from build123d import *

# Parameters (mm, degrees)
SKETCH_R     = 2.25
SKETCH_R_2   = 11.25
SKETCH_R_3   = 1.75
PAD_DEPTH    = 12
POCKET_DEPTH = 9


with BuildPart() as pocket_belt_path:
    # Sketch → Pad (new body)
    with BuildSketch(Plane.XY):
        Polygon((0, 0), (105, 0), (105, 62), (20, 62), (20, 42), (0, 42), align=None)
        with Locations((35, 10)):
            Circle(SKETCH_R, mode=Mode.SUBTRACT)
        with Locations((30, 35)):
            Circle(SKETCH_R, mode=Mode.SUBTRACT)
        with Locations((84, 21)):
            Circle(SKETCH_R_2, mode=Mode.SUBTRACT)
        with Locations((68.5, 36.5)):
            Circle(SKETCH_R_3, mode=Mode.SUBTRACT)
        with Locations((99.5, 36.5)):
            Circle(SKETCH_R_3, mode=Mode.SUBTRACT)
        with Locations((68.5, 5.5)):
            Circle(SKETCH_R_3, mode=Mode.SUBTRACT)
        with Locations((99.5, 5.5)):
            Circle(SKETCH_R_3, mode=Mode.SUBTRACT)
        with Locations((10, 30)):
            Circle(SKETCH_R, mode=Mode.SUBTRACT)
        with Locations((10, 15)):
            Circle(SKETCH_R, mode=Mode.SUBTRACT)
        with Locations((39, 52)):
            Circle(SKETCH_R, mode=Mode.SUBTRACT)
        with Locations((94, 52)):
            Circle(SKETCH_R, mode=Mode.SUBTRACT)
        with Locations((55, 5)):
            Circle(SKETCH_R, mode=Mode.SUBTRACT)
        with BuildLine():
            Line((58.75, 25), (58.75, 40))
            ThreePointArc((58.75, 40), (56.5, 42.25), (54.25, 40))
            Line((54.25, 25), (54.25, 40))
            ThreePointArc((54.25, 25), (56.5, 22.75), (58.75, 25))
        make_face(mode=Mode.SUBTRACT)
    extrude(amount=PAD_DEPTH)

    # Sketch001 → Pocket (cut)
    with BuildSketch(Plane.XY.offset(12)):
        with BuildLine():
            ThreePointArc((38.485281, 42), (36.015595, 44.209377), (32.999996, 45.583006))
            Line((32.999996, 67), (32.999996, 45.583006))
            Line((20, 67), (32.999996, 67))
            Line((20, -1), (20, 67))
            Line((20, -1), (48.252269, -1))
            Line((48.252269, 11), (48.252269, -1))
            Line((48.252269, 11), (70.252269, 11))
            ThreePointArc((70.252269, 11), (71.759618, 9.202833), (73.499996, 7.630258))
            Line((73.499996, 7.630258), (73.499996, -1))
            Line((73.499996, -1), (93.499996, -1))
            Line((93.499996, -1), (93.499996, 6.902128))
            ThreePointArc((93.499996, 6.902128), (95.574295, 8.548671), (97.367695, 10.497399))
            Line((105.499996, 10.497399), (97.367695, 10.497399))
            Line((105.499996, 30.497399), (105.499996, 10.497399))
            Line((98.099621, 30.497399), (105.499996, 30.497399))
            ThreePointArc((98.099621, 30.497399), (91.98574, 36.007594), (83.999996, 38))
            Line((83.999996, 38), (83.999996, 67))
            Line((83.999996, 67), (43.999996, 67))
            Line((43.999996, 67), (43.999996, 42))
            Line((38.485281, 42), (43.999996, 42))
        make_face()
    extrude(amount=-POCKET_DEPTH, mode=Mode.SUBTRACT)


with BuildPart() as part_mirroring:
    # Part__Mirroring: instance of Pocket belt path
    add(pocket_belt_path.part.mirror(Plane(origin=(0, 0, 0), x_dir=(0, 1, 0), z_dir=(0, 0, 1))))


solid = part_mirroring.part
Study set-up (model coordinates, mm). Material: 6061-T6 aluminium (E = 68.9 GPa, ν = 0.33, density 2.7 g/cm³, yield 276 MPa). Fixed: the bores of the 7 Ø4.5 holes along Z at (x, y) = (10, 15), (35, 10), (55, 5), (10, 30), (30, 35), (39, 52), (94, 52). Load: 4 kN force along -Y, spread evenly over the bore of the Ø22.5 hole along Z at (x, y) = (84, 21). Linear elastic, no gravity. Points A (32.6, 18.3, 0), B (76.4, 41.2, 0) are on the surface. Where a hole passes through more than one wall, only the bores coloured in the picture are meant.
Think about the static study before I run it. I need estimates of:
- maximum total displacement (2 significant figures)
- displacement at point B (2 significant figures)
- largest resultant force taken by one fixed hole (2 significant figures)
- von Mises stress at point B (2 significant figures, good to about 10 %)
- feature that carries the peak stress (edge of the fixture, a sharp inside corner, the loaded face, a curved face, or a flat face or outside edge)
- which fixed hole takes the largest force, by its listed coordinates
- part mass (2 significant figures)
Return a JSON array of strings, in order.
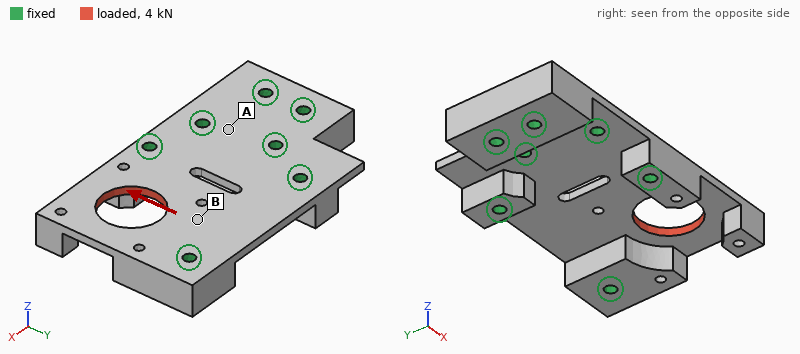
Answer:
["31 µm", "7.7 µm", "2.5 kN", "12 MPa", "the loaded face", "(94, 52)", "91 g"]
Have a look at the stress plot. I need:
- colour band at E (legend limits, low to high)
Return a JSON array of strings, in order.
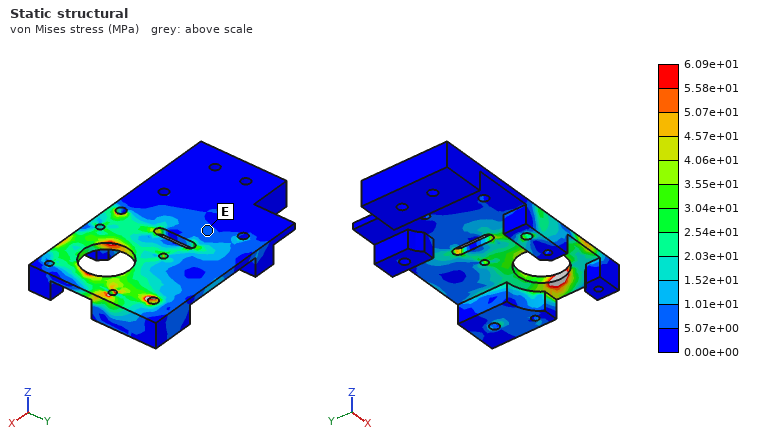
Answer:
["5.07e+00 to 1.01e+01 MPa"]
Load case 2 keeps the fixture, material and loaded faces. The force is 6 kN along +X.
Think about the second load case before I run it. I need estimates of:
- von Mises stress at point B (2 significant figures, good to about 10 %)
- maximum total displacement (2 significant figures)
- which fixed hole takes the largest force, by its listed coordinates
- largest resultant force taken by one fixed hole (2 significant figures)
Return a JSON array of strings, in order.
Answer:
["30 MPa", "47 µm", "(55, 5)", "2.6 kN"]
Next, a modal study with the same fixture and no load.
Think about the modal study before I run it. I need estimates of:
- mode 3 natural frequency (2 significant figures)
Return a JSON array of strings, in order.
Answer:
["7900 Hz"]
